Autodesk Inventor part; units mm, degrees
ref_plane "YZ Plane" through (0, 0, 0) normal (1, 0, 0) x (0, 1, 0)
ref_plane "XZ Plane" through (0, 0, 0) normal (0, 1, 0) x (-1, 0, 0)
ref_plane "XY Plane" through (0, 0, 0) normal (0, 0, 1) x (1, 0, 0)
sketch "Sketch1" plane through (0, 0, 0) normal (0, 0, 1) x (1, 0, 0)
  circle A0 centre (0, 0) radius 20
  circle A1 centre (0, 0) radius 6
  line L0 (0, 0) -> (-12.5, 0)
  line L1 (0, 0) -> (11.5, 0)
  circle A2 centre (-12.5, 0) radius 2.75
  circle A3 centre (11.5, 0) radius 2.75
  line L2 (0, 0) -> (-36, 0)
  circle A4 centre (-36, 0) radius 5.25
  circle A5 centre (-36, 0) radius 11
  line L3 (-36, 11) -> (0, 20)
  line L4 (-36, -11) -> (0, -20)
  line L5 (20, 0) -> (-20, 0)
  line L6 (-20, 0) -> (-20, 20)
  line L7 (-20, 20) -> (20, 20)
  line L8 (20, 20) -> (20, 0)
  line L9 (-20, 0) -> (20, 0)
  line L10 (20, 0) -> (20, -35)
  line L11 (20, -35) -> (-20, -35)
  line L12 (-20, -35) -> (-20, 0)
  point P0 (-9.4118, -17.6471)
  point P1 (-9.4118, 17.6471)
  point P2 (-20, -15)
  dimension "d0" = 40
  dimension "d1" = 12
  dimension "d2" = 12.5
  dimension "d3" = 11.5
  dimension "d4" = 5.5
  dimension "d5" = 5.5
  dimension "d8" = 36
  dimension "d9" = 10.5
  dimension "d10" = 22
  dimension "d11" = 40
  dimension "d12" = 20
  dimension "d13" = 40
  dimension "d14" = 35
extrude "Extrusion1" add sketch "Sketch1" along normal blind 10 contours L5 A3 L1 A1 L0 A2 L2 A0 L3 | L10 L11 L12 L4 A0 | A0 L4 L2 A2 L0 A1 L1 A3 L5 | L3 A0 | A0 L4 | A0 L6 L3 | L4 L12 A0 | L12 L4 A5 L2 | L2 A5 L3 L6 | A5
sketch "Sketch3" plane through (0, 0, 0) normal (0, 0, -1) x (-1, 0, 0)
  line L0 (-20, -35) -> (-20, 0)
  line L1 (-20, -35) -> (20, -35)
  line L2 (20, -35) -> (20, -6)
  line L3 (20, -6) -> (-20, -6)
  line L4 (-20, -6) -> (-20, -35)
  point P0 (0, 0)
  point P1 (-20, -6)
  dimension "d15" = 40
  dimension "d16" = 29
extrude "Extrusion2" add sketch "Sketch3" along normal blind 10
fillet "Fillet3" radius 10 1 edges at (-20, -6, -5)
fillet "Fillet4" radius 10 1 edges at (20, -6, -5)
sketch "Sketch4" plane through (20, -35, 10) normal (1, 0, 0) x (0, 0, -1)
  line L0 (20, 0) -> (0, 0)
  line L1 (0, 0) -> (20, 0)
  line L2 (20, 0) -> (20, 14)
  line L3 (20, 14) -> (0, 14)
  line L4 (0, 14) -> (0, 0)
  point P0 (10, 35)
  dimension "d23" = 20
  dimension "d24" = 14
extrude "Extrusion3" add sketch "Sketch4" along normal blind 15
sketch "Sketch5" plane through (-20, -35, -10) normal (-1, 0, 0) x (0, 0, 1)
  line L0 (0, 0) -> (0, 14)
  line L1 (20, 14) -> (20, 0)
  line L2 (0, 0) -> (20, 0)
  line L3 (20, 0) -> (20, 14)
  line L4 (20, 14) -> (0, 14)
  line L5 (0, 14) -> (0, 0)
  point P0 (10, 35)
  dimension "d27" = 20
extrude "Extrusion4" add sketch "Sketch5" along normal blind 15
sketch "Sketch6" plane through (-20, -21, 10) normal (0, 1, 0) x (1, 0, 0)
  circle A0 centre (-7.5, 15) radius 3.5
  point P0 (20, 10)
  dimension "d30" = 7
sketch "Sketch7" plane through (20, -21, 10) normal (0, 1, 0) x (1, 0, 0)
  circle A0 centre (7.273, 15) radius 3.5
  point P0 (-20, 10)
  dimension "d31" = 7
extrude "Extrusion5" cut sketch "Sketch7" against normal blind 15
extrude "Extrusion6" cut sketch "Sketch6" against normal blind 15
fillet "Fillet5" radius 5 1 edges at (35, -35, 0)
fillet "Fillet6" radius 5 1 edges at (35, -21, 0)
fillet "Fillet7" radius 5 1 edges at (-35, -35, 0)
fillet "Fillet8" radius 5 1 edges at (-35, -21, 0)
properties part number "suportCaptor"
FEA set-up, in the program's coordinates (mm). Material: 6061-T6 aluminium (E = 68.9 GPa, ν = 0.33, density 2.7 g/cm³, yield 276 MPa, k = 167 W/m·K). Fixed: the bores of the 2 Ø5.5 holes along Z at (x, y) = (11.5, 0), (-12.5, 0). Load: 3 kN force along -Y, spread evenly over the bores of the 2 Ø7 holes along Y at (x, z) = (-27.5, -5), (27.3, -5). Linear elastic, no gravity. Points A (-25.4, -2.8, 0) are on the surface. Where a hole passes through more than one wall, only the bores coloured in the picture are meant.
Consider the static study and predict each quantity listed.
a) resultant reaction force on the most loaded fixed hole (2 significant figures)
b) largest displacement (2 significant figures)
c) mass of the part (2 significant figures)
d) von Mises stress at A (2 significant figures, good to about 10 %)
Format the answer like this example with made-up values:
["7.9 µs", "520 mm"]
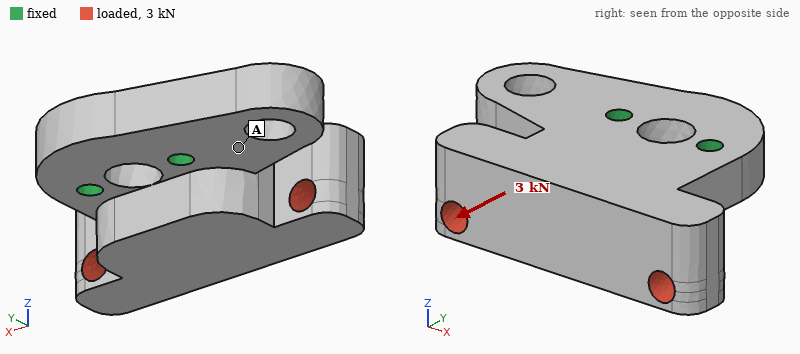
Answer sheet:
["1.5 kN", "65 µm", "110 g", "12 MPa"]
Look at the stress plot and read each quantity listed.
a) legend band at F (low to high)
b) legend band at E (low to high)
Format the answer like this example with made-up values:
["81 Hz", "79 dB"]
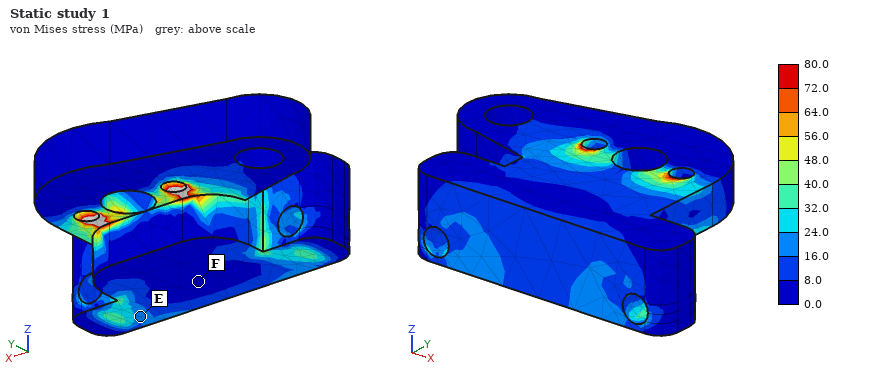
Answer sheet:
["0.0 to 8.0 MPa", "16.0 to 24.0 MPa"]
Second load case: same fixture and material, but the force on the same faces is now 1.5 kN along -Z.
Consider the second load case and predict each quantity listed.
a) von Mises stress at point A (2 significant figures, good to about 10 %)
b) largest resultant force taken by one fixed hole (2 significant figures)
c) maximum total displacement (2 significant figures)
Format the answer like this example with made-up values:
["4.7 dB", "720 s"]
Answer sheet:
["14 MPa", "770 N", "70 µm"]
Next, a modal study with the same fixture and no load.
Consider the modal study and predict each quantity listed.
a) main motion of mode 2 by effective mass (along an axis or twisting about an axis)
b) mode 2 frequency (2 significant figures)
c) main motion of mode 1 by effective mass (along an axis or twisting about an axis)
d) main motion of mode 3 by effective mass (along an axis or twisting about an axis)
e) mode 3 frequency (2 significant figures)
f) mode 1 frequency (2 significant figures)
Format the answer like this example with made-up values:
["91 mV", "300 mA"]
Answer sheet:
["twisting about Y", "7200 Hz", "along Z", "along X", "8400 Hz", "3700 Hz"]
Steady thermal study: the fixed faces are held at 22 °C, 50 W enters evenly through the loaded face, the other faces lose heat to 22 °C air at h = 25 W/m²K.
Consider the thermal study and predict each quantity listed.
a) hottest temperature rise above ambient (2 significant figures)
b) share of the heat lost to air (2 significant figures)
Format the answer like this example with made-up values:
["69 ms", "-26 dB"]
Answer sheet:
["25 K", "5.0 %"]
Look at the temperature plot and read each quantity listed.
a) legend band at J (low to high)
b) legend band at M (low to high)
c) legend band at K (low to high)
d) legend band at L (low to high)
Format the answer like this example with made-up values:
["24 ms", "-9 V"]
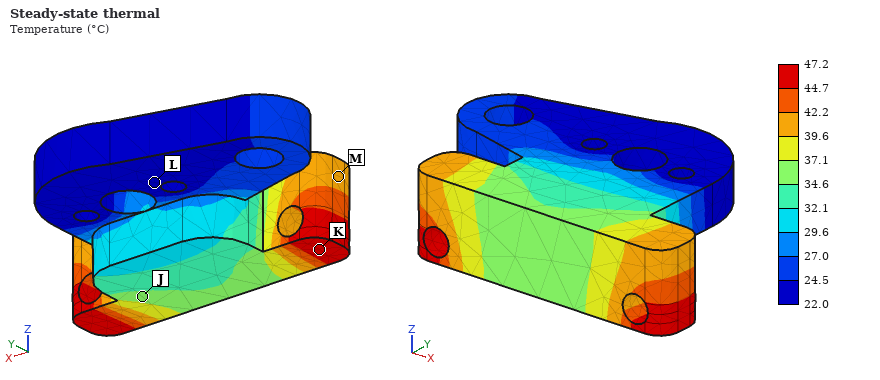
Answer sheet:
["34.6 to 37.1 °C", "39.6 to 42.2 °C", "44.7 to 47.2 °C", "22.0 to 24.5 °C"]
